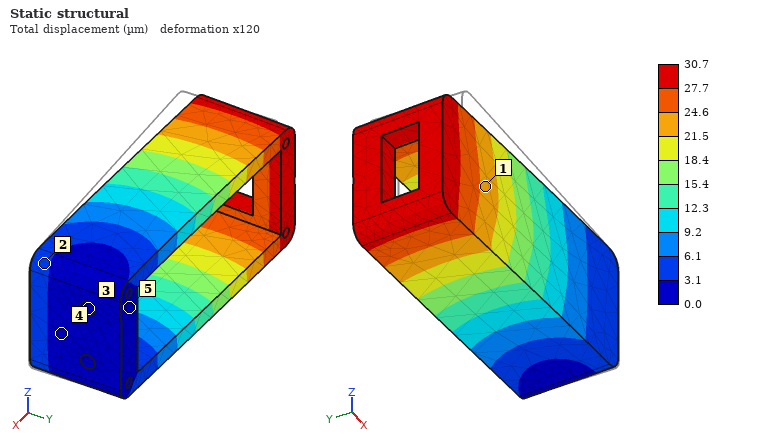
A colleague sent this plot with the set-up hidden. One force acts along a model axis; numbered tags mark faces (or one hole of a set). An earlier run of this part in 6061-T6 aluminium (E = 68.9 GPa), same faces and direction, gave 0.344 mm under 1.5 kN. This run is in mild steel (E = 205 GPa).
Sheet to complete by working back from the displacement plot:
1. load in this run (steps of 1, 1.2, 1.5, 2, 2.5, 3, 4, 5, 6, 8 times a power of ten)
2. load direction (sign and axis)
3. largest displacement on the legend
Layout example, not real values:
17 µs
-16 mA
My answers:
400 N
+Y
30.7 µm
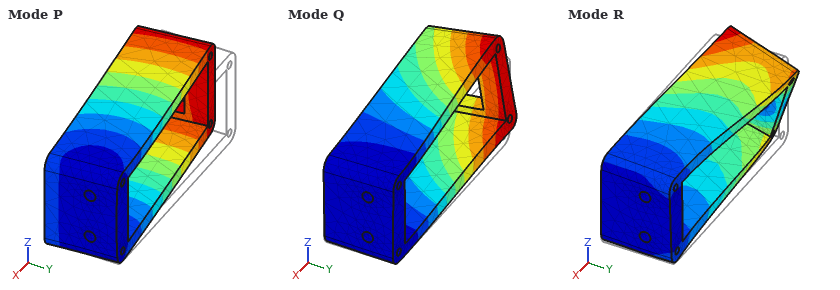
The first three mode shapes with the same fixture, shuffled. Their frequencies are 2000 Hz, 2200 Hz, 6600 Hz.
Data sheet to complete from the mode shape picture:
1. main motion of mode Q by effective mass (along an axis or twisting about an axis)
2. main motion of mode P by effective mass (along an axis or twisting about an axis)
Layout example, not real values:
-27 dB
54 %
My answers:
along Z
along Y
